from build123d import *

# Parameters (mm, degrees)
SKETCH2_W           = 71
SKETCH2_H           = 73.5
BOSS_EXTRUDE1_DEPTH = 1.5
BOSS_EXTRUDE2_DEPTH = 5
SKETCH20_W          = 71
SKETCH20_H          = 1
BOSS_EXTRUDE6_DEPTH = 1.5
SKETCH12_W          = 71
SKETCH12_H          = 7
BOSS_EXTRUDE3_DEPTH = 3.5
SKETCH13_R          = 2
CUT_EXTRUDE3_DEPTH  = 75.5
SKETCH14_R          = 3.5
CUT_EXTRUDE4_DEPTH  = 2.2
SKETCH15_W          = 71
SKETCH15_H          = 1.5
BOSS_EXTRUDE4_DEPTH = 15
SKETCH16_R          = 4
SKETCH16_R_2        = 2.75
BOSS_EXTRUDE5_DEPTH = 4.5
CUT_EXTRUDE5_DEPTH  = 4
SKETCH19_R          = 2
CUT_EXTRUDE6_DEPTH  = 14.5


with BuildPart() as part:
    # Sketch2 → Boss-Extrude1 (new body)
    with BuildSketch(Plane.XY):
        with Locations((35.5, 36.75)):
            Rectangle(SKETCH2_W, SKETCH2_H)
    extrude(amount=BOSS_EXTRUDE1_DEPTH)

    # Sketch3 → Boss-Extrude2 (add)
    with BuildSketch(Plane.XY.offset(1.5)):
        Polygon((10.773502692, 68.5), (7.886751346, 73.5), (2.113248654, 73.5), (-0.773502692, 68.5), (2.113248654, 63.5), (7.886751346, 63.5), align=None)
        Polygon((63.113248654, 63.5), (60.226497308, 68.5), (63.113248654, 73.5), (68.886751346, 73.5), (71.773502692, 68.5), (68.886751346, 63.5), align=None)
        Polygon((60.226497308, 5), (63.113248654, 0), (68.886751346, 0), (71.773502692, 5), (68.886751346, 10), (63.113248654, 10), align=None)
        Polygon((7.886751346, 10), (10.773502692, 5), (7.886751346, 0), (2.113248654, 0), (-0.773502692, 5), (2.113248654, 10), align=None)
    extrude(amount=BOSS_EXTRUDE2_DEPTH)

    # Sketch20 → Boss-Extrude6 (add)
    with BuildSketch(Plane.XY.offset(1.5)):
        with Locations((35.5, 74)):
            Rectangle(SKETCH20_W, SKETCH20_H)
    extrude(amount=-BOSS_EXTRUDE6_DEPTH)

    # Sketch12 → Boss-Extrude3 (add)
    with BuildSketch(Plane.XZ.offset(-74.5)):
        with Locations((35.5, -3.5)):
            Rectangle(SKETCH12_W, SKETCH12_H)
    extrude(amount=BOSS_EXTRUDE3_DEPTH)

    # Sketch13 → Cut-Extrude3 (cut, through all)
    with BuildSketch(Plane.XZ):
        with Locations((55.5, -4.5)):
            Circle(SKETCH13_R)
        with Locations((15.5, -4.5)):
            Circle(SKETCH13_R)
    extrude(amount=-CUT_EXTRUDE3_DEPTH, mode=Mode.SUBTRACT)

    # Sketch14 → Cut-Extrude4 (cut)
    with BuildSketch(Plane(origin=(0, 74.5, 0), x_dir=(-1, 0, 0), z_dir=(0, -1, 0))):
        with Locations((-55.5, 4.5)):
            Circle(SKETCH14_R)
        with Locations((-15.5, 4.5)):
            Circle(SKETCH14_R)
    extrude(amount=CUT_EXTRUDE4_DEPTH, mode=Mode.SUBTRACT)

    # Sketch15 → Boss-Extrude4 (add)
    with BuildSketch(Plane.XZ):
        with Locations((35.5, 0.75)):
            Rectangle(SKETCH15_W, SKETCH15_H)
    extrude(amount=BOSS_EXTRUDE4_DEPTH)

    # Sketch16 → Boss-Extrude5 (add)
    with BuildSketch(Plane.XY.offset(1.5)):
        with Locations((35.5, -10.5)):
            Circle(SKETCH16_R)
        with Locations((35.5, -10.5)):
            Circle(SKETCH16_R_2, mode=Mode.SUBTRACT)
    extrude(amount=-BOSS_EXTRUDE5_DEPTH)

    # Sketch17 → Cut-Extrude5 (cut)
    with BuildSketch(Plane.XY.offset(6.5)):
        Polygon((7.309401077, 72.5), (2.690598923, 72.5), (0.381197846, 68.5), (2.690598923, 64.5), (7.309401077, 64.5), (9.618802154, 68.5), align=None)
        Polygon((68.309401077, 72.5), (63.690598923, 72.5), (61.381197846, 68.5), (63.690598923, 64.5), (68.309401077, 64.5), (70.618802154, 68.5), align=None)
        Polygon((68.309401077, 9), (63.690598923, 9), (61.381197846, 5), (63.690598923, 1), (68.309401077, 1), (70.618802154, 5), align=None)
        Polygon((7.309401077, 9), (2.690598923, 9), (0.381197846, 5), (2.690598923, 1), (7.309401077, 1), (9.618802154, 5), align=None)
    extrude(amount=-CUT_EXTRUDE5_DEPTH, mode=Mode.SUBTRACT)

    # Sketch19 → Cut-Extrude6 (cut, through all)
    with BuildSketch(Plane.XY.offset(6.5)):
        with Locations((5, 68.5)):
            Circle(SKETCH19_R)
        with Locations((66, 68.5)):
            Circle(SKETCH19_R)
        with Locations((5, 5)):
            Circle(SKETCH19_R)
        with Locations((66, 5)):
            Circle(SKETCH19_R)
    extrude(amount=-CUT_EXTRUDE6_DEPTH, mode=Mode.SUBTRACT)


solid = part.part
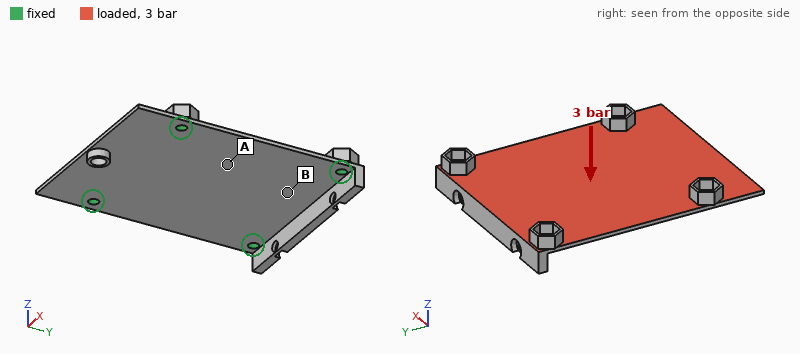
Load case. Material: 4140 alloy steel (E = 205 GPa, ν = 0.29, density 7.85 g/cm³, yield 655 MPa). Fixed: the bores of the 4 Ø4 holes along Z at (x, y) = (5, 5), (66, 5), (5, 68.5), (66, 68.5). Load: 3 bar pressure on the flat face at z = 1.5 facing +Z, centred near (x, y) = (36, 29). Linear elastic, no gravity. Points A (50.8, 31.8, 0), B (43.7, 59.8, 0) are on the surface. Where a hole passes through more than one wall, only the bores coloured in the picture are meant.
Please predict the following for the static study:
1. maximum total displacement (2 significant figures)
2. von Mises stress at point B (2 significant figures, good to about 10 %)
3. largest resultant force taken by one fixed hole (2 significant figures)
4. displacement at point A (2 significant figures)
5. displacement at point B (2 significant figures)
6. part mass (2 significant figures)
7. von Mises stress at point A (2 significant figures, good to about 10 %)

0.32 mm
55 MPa
590 N
0.27 mm
0.12 mm
93 g
120 MPa
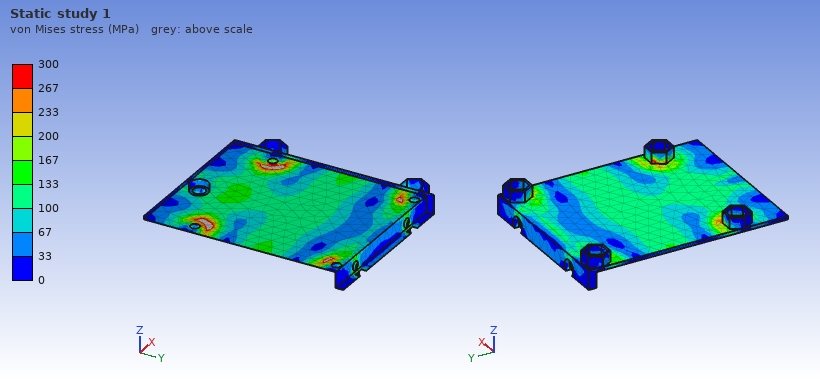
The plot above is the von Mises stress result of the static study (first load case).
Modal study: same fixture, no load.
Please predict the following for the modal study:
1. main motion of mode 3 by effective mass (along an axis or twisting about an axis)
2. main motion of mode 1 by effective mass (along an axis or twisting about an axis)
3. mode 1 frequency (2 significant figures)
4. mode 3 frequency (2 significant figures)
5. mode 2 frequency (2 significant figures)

twisting about Y
along Z
1700 Hz
2700 Hz
2000 Hz
